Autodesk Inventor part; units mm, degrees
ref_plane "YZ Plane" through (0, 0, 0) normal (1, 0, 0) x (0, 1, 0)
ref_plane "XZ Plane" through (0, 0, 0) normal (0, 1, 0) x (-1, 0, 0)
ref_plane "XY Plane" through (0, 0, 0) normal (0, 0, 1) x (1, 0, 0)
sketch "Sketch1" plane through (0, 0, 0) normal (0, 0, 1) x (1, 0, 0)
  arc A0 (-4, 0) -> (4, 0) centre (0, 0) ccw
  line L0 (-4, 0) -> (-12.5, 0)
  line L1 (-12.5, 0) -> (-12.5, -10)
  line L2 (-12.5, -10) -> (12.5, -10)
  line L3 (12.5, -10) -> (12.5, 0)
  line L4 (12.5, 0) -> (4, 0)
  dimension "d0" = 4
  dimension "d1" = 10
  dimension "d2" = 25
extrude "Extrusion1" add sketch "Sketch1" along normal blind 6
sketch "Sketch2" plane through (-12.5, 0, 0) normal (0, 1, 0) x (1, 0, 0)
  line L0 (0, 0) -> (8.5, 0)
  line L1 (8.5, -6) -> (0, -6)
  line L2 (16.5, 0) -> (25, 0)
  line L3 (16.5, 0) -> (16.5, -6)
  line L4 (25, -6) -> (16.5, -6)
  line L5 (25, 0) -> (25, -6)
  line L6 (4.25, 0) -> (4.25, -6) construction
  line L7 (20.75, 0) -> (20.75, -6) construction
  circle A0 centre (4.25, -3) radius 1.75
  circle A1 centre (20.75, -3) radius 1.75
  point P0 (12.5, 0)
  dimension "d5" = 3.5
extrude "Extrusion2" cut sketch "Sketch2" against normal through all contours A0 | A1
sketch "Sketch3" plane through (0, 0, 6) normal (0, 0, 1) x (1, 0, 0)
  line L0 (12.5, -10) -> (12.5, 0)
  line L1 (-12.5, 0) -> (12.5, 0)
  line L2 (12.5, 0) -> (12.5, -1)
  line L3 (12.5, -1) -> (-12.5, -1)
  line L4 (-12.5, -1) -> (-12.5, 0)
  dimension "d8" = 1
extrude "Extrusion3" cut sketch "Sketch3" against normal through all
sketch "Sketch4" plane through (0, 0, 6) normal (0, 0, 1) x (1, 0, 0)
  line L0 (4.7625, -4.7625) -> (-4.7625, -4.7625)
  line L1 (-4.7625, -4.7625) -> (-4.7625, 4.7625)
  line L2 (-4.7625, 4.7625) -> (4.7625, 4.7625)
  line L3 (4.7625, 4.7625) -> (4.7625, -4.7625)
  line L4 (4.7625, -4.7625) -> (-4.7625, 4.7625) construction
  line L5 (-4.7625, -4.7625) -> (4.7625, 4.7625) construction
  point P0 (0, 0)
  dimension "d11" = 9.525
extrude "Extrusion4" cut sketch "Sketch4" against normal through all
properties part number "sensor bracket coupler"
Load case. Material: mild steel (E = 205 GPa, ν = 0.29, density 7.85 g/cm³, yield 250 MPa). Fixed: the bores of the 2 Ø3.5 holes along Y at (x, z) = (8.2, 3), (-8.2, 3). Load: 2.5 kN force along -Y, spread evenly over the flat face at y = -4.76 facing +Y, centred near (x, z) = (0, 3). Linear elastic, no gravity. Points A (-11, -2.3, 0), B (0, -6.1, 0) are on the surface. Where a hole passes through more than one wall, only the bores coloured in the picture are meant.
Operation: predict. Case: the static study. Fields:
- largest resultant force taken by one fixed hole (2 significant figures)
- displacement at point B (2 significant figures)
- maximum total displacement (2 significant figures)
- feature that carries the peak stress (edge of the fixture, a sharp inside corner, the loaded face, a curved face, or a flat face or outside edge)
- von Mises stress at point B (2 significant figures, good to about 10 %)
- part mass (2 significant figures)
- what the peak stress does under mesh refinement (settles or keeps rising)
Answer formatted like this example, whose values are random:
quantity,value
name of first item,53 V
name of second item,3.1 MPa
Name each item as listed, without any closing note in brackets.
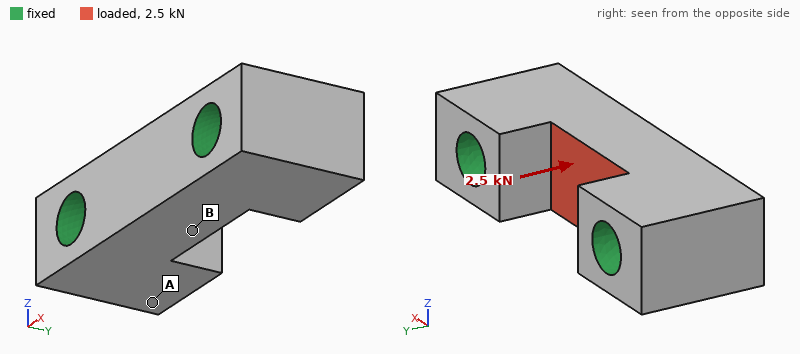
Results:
quantity,value
largest resultant force taken by one fixed hole,1.3 kN
displacement at point B,3.6 µm
maximum total displacement,3.8 µm
feature that carries the peak stress,edge of the fixture
von Mises stress at point B,33 MPa
part mass,7.6 g
what the peak stress does under mesh refinement,keeps rising
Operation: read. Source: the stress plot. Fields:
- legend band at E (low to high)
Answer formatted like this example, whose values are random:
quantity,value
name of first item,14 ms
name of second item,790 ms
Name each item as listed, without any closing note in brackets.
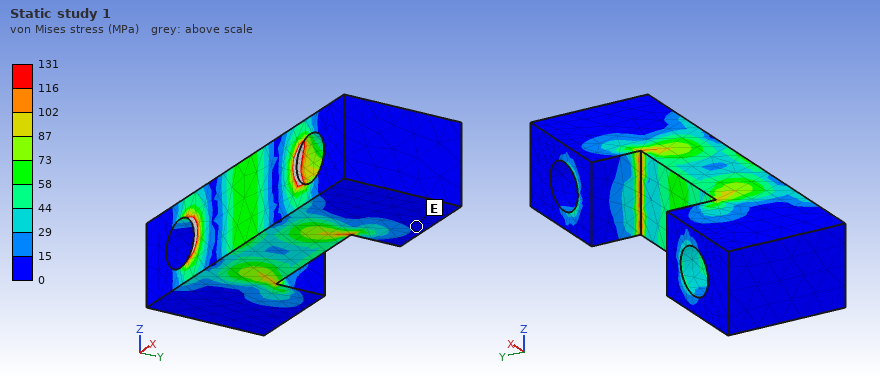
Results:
quantity,value
legend band at E,0 to 15 MPa
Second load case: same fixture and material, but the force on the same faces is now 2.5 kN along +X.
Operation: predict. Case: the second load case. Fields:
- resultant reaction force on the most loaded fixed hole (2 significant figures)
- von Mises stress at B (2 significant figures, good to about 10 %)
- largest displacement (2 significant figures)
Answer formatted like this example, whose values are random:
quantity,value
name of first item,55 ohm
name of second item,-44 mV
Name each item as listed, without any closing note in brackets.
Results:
quantity,value
resultant reaction force on the most loaded fixed hole,1.3 kN
von Mises stress at B,36 MPa
largest displacement,1.9 µm
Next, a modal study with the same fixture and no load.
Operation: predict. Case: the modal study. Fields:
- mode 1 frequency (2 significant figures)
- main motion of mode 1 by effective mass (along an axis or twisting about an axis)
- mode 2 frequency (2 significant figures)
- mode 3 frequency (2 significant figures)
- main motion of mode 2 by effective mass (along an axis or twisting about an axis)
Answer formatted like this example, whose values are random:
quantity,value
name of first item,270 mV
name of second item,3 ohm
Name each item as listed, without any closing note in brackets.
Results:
quantity,value
mode 1 frequency,85 kHz
main motion of mode 1 by effective mass,along Z
mode 2 frequency,96 kHz
mode 3 frequency,120 kHz
main motion of mode 2 by effective mass,along Y
